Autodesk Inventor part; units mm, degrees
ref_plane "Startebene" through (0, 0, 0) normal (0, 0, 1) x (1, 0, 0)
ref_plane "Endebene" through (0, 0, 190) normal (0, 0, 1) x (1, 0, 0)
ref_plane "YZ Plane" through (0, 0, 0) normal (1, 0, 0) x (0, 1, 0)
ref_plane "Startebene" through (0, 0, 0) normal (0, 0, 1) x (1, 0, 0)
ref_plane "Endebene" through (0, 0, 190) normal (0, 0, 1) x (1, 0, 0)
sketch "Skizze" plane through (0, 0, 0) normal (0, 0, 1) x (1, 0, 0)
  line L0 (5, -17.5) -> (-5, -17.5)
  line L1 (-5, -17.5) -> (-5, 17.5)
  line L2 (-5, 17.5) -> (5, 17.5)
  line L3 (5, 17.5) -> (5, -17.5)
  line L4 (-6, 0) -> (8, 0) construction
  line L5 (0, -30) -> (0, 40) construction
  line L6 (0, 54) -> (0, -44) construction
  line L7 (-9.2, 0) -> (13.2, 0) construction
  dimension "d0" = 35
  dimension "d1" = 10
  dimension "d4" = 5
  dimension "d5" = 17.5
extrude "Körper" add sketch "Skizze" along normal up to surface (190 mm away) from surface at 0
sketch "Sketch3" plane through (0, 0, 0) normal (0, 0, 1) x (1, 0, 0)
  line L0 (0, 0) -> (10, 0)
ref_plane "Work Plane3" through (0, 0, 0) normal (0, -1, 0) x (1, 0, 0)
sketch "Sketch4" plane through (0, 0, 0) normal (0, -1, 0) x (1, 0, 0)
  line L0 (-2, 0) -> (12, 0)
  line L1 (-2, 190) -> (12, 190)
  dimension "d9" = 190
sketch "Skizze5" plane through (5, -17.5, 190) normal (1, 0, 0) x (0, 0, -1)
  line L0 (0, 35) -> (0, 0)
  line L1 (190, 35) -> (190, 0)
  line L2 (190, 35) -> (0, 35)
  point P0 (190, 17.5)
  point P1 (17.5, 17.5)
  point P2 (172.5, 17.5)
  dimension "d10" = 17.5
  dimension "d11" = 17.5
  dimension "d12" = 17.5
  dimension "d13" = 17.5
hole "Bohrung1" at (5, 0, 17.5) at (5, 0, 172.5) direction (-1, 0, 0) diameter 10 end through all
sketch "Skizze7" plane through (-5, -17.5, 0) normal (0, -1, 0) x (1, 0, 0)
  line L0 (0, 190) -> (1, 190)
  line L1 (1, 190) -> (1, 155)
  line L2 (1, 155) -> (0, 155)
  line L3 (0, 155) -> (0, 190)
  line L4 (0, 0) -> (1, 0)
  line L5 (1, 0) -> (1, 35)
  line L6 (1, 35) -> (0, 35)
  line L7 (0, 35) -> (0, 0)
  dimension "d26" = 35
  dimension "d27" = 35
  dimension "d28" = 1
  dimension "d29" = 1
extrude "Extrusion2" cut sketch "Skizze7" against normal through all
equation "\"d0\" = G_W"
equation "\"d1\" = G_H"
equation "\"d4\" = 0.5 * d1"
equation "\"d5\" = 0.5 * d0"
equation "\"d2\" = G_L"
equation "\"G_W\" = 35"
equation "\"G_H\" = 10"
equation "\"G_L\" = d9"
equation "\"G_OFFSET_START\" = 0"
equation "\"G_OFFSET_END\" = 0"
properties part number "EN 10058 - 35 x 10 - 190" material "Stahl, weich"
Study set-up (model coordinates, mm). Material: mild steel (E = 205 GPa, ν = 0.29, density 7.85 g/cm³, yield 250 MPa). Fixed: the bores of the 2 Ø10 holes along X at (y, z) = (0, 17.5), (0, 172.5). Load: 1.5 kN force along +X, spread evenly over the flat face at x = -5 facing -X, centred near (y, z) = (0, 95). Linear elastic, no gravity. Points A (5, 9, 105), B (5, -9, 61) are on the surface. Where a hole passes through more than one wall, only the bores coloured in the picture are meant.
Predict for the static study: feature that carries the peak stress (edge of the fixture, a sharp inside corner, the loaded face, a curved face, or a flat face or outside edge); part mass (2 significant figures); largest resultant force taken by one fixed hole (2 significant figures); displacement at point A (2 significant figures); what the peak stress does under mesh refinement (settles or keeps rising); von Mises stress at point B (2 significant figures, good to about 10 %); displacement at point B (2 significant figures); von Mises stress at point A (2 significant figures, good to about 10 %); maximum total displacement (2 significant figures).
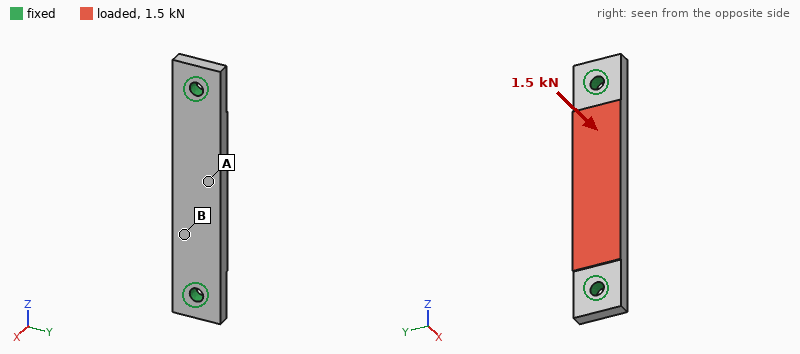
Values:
edge of the fixture
490 g
790 N
33 µm
keeps rising
9.3 MPa
23 µm
20 MPa
35 µm
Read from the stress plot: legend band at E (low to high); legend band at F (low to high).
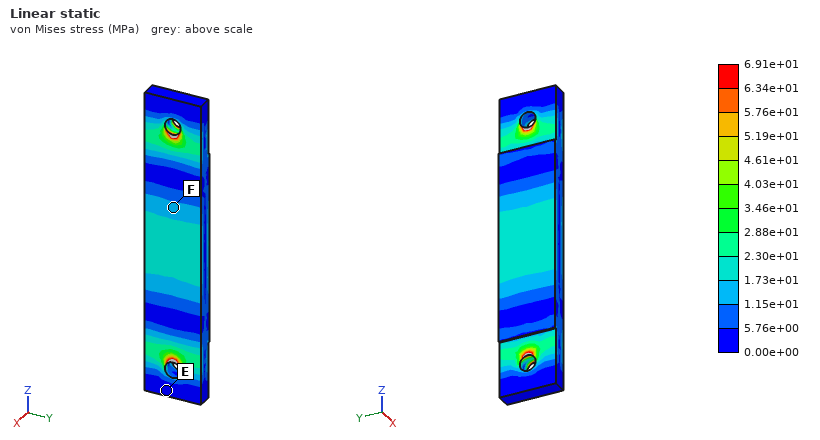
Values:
0.00e+00 to 5.76e+00 MPa
1.15e+01 to 1.73e+01 MPa
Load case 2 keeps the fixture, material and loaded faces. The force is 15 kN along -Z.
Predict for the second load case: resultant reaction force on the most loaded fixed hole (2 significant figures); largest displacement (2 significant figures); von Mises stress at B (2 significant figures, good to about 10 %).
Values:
7.5 kN
5.9 µm
11 MPa
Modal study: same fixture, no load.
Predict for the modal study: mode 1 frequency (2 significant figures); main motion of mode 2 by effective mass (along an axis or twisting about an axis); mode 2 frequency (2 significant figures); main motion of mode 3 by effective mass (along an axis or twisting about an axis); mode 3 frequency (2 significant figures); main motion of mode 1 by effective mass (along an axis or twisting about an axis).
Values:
2100 Hz
along Y
4700 Hz
twisting about Z
5100 Hz
along X
